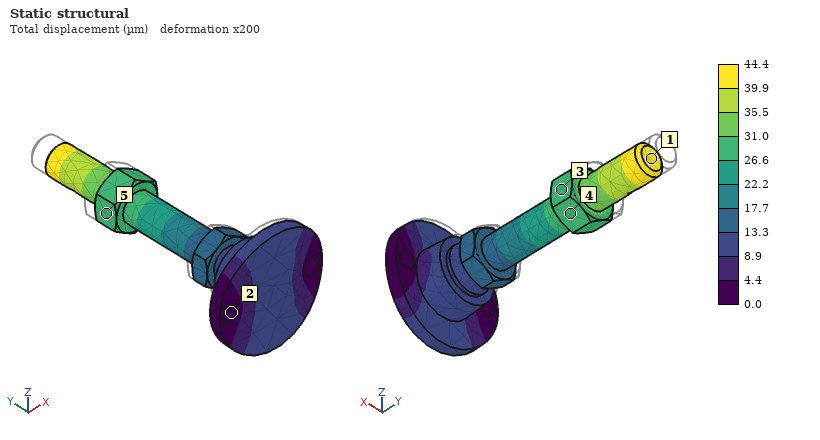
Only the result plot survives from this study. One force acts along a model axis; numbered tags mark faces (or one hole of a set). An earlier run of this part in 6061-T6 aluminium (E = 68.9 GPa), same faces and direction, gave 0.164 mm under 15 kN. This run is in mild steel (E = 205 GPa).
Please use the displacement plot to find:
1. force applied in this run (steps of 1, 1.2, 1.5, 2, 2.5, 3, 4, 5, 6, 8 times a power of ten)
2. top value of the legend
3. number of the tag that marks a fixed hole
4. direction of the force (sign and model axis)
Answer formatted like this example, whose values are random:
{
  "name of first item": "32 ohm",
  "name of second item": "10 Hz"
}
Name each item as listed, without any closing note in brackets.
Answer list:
{
  "force applied in this run": "12 kN",
  "top value of the legend": "44.4 µm",
  "number of the tag that marks a fixed hole": "2",
  "direction of the force": "-Y"
}
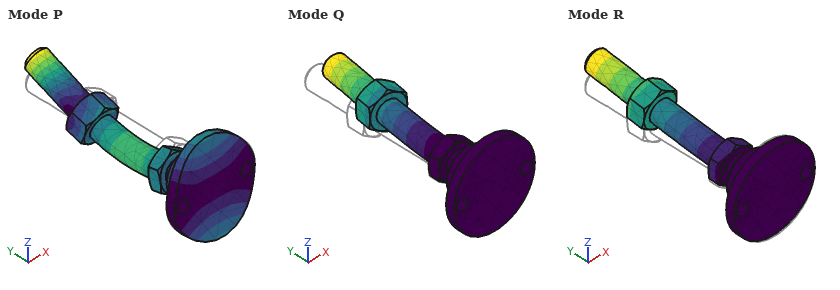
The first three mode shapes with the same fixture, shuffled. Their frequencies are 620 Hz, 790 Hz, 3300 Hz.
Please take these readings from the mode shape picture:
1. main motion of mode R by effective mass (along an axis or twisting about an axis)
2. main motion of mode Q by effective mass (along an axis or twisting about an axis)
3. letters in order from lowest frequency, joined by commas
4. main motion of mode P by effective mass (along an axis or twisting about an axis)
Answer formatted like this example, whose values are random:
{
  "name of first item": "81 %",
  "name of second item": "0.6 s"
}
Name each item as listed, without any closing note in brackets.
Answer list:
{
  "main motion of mode R by effective mass": "along Z",
  "main motion of mode Q by effective mass": "along X",
  "letters in order from lowest frequency, joined by commas": "R, Q, P",
  "main motion of mode P by effective mass": "along Z"
}
